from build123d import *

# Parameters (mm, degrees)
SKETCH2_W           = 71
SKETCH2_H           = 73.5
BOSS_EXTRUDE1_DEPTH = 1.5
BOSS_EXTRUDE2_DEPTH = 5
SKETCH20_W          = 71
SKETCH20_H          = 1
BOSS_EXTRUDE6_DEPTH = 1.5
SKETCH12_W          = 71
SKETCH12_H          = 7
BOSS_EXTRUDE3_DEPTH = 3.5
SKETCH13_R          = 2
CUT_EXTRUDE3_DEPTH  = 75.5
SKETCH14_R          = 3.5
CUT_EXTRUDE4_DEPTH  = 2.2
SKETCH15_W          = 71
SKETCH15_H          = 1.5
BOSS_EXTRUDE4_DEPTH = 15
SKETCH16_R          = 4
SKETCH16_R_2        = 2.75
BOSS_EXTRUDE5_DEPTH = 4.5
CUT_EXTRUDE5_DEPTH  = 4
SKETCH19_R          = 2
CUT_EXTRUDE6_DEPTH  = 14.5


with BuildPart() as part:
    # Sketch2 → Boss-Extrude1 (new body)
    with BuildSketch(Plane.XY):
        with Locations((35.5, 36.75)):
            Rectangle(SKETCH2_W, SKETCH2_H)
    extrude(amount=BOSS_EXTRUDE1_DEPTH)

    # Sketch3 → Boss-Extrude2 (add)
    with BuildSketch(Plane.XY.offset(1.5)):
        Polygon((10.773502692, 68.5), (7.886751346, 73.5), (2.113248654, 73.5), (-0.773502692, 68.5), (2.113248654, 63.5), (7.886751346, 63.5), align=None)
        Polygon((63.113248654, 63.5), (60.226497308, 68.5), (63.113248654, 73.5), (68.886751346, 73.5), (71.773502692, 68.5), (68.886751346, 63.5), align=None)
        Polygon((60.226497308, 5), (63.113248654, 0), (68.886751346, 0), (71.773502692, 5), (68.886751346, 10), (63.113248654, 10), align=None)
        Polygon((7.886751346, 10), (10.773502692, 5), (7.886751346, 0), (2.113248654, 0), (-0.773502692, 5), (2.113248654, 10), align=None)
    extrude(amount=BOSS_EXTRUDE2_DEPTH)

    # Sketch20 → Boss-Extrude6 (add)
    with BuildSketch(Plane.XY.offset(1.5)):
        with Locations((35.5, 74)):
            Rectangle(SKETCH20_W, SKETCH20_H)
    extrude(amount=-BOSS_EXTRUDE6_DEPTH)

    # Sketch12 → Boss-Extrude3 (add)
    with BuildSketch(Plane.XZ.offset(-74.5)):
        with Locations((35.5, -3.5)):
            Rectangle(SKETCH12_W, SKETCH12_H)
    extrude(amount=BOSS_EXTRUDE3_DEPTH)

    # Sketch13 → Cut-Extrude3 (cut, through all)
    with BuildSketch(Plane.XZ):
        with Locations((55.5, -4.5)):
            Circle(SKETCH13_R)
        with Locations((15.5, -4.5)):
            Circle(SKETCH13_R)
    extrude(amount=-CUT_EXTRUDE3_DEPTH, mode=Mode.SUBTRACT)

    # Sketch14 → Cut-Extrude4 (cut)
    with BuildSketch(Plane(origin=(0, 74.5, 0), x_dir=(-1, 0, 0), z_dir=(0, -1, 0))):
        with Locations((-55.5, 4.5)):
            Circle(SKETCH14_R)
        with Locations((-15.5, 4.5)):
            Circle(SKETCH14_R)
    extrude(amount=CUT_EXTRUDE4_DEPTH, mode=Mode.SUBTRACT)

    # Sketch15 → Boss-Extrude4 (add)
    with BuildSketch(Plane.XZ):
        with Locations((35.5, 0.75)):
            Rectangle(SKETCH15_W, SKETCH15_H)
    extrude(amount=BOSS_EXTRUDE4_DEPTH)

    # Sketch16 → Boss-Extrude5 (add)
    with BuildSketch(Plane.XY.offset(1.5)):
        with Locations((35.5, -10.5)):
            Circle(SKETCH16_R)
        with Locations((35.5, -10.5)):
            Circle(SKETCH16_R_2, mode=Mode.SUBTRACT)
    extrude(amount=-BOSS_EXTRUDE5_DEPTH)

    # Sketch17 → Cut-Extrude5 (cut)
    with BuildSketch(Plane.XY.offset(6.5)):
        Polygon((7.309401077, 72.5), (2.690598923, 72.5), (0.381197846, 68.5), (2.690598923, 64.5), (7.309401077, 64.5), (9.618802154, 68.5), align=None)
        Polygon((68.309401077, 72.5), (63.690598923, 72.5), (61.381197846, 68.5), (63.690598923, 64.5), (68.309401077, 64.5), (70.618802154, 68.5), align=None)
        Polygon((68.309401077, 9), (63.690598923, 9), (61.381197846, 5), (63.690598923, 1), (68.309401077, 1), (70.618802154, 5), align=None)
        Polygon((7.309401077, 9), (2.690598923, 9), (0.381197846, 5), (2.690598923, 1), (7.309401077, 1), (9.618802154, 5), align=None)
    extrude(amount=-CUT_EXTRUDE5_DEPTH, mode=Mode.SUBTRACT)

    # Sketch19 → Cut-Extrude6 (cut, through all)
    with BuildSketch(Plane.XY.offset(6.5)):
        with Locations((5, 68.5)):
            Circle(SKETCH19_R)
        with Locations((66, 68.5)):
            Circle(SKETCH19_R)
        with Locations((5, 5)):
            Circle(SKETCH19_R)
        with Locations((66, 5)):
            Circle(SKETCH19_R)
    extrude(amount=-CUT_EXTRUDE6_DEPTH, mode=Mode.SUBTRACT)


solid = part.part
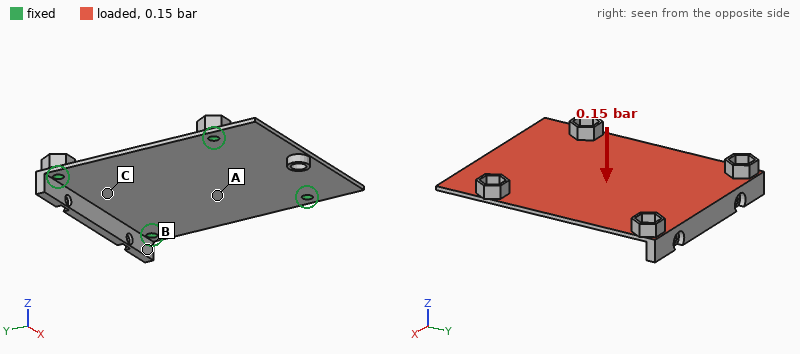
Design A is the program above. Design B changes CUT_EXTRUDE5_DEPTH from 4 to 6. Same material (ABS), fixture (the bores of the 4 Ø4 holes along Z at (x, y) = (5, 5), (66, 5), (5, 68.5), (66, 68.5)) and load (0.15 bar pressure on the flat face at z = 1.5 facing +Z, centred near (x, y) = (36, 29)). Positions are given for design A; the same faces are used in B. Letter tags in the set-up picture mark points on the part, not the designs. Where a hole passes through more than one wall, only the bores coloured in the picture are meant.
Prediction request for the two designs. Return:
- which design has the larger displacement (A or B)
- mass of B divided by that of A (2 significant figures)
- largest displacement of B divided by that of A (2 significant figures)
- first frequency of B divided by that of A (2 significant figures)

B
0.97
1.6
0.75
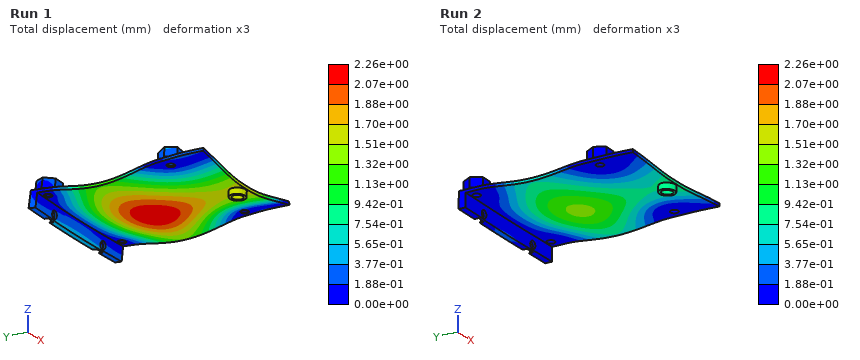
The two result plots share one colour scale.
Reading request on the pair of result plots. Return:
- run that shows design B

Run 1
